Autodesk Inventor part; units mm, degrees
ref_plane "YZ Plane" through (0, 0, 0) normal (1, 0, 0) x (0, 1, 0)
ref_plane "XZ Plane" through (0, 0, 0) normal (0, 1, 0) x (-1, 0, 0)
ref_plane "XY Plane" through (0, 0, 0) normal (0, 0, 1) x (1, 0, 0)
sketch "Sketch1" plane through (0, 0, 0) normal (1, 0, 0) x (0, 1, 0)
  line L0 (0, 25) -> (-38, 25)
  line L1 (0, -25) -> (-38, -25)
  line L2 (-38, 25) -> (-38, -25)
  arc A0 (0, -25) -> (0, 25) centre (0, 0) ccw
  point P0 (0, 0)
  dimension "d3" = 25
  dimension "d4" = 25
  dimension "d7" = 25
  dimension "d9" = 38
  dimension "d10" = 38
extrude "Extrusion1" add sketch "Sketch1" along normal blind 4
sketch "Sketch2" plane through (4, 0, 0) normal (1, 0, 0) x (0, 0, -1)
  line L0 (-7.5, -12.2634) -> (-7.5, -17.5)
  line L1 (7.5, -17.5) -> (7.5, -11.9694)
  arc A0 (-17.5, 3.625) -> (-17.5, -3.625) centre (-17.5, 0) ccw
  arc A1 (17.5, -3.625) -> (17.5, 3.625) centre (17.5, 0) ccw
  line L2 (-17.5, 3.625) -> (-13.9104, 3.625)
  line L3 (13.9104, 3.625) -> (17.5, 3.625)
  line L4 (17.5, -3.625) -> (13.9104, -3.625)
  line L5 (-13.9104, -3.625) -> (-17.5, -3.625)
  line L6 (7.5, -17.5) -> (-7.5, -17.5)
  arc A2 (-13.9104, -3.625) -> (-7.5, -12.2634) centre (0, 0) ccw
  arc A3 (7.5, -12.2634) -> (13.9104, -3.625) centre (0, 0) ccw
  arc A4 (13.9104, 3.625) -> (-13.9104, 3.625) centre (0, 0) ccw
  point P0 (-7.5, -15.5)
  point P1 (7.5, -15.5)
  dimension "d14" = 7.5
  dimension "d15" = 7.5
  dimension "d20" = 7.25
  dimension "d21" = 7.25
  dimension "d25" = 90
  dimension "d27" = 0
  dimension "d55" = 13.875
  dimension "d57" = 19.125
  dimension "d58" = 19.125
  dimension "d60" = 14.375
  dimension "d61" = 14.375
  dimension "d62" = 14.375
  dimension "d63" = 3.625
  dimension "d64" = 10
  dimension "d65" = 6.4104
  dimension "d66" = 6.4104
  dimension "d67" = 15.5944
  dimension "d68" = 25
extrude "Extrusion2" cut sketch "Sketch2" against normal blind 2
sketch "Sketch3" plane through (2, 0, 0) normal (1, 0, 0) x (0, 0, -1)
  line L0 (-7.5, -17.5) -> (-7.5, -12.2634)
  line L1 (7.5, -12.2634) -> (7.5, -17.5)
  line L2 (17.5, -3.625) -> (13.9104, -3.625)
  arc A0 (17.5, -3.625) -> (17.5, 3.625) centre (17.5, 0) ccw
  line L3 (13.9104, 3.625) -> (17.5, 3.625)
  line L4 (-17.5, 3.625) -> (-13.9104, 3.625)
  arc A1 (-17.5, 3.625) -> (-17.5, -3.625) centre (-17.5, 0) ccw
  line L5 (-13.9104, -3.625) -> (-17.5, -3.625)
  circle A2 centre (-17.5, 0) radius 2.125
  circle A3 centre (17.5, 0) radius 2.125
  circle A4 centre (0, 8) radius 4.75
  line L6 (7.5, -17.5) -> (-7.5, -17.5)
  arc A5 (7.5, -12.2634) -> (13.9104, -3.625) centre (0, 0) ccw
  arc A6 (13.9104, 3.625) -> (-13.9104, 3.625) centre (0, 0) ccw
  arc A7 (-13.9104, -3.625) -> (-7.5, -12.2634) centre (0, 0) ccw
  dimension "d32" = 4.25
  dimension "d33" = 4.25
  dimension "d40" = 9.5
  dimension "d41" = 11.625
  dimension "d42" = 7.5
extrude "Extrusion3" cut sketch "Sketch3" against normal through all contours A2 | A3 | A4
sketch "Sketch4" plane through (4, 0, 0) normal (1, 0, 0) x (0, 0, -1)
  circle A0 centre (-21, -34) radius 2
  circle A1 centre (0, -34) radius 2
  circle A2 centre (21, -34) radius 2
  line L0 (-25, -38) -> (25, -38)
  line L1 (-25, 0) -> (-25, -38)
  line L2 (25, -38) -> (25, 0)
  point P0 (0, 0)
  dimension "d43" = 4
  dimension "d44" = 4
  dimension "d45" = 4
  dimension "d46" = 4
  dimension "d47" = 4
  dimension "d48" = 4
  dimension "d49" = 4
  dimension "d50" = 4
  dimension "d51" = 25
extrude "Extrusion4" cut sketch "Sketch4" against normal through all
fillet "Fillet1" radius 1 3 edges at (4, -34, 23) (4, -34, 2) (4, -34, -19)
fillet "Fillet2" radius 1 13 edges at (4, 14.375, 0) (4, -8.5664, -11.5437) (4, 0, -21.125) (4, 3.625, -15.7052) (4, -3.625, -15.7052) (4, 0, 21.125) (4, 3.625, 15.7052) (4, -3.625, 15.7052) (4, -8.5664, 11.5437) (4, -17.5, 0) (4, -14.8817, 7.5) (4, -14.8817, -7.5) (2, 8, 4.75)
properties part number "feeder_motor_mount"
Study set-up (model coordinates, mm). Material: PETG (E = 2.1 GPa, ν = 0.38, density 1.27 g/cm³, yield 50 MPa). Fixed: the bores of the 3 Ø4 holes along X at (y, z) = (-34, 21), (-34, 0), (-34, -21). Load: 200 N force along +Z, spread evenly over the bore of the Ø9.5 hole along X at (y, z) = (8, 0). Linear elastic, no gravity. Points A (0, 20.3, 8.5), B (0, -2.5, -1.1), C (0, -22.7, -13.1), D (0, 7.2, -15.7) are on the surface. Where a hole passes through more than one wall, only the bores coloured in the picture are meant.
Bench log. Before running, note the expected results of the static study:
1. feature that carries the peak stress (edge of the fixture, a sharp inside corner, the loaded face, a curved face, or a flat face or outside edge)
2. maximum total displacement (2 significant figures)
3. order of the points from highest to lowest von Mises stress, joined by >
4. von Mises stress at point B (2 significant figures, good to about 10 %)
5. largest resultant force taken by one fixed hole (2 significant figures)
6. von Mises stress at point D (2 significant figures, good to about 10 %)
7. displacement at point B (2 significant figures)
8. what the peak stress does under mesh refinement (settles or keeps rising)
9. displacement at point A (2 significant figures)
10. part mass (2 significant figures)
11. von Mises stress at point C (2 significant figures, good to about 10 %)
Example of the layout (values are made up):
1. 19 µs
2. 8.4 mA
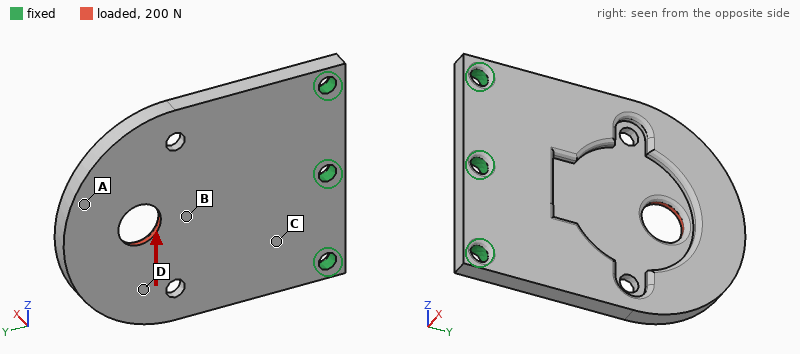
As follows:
1. edge of the fixture
2. 0.23 mm
3. B > C > D > A
4. 6.5 MPa
5. 200 N
6. 2.5 MPa
7. 0.11 mm
8. keeps rising
9. 0.22 mm
10. 12 g
11. 3.2 MPa
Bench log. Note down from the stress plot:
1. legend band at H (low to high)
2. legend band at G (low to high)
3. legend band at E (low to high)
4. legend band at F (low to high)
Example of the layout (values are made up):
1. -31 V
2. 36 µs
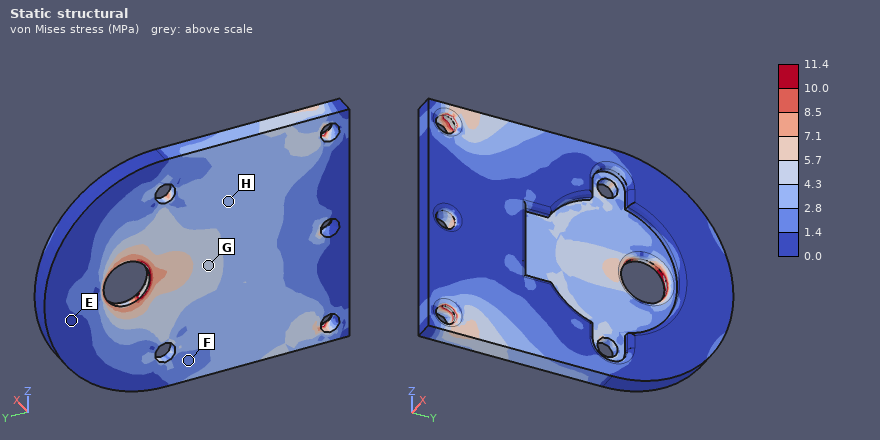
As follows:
1. 2.8 to 4.3 MPa
2. 4.3 to 5.7 MPa
3. 0.0 to 1.4 MPa
4. 1.4 to 2.8 MPa
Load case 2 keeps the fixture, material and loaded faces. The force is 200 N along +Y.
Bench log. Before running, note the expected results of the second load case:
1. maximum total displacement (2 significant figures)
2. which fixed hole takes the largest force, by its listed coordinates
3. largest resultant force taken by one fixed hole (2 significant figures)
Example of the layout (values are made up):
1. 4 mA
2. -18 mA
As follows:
1. 0.92 mm
2. (-34, 0)
3. 75 N
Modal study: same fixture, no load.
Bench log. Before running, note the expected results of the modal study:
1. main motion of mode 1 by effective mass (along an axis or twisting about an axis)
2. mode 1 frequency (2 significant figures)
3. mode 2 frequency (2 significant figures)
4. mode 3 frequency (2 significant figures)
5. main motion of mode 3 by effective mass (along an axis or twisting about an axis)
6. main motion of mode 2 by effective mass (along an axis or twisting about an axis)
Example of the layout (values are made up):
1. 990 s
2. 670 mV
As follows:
1. along X
2. 270 Hz
3. 720 Hz
4. 1200 Hz
5. along X
6. twisting about Y
